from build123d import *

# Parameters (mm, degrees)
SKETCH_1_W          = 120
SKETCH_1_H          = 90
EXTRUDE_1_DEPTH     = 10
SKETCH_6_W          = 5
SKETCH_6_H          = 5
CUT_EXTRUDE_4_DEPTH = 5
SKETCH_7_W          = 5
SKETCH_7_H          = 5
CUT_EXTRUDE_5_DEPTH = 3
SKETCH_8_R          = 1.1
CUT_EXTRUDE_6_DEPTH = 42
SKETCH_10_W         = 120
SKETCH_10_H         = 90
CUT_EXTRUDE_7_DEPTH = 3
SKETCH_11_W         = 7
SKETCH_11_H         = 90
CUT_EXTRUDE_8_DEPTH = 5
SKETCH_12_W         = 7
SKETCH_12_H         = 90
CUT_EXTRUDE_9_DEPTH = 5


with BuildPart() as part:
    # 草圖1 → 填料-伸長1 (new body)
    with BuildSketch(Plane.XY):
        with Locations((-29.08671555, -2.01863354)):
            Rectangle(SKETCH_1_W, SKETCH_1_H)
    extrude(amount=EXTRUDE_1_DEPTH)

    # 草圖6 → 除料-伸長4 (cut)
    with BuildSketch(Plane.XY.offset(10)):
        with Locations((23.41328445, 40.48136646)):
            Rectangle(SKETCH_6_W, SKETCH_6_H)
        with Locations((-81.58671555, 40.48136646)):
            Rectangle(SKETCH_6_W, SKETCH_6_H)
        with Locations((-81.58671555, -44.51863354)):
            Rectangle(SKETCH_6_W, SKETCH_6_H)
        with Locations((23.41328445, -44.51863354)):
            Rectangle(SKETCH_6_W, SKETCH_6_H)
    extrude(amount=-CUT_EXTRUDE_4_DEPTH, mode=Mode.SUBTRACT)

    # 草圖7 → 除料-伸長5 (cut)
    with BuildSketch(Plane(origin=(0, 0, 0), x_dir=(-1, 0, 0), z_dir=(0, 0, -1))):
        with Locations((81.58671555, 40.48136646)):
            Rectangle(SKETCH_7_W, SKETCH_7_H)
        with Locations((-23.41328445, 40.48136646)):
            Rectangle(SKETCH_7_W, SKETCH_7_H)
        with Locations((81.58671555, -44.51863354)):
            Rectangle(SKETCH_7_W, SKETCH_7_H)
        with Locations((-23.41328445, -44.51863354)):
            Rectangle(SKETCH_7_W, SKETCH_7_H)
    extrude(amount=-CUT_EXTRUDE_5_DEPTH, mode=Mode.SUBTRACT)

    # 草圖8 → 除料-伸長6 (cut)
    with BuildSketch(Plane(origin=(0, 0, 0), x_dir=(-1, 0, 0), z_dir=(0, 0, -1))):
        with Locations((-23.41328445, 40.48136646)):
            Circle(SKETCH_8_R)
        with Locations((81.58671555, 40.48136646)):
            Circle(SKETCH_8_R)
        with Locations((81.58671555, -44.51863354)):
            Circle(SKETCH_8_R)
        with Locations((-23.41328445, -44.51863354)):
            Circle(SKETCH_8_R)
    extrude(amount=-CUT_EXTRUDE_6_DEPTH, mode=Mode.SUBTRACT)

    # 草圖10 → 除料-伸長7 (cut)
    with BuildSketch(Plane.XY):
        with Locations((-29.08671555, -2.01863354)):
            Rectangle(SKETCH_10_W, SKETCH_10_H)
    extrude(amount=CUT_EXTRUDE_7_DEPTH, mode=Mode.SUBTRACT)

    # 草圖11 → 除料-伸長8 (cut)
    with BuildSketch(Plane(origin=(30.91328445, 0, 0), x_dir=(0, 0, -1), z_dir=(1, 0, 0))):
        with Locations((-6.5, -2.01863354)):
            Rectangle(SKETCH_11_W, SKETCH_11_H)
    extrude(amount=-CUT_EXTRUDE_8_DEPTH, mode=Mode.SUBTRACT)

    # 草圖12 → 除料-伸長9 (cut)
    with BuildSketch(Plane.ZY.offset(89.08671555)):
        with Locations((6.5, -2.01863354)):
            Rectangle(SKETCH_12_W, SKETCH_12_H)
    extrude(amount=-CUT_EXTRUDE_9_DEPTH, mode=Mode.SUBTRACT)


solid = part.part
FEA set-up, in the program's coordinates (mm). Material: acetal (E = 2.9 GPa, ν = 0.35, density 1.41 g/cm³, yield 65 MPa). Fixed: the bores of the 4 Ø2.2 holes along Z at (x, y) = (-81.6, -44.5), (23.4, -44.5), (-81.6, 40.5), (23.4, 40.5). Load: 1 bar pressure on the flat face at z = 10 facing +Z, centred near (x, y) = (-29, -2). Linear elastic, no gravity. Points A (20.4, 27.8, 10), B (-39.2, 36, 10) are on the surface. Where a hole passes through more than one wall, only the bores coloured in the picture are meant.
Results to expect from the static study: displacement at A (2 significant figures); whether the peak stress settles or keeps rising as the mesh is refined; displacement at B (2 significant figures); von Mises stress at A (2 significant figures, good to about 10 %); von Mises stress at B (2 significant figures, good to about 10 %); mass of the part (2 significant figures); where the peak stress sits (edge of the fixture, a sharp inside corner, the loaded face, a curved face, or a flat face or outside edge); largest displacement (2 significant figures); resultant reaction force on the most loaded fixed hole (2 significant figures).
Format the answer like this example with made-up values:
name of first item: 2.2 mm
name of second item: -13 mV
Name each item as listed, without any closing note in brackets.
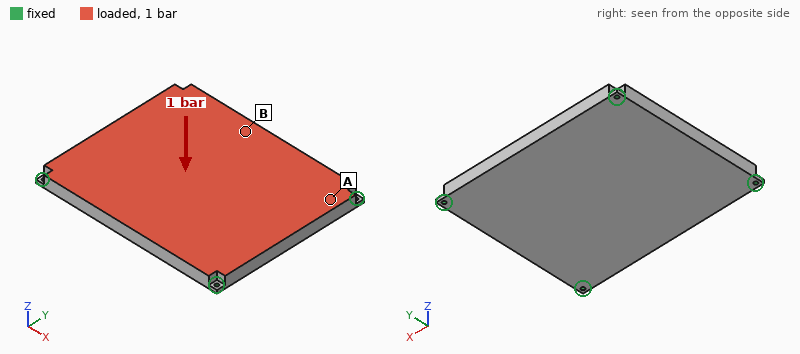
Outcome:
displacement at A: 0.40 mm
whether the peak stress settles or keeps rising as the mesh is refined: keeps rising
displacement at B: 1.4 mm
von Mises stress at A: 7.2 MPa
von Mises stress at B: 14 MPa
mass of the part: 97 g
where the peak stress sits: edge of the fixture
largest displacement: 1.6 mm
resultant reaction force on the most loaded fixed hole: 600 N
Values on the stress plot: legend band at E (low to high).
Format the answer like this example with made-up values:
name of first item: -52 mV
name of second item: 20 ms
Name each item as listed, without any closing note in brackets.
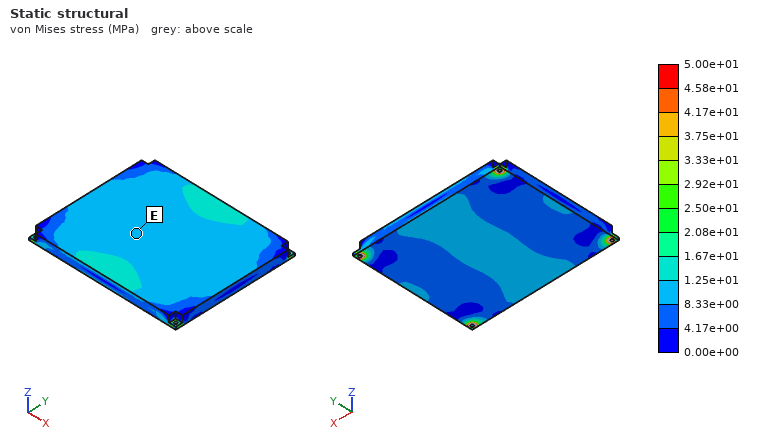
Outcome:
legend band at E: 8.33e+00 to 1.25e+01 MPa
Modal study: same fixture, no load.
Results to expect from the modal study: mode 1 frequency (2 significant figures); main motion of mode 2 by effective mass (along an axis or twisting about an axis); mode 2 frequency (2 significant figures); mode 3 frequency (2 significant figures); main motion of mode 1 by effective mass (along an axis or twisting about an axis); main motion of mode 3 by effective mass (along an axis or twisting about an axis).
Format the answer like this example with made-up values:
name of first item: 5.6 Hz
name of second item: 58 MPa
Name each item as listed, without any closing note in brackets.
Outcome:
mode 1 frequency: 460 Hz
main motion of mode 2 by effective mass: twisting about X
mode 2 frequency: 830 Hz
mode 3 frequency: 970 Hz
main motion of mode 1 by effective mass: along Z
main motion of mode 3 by effective mass: twisting about Y
